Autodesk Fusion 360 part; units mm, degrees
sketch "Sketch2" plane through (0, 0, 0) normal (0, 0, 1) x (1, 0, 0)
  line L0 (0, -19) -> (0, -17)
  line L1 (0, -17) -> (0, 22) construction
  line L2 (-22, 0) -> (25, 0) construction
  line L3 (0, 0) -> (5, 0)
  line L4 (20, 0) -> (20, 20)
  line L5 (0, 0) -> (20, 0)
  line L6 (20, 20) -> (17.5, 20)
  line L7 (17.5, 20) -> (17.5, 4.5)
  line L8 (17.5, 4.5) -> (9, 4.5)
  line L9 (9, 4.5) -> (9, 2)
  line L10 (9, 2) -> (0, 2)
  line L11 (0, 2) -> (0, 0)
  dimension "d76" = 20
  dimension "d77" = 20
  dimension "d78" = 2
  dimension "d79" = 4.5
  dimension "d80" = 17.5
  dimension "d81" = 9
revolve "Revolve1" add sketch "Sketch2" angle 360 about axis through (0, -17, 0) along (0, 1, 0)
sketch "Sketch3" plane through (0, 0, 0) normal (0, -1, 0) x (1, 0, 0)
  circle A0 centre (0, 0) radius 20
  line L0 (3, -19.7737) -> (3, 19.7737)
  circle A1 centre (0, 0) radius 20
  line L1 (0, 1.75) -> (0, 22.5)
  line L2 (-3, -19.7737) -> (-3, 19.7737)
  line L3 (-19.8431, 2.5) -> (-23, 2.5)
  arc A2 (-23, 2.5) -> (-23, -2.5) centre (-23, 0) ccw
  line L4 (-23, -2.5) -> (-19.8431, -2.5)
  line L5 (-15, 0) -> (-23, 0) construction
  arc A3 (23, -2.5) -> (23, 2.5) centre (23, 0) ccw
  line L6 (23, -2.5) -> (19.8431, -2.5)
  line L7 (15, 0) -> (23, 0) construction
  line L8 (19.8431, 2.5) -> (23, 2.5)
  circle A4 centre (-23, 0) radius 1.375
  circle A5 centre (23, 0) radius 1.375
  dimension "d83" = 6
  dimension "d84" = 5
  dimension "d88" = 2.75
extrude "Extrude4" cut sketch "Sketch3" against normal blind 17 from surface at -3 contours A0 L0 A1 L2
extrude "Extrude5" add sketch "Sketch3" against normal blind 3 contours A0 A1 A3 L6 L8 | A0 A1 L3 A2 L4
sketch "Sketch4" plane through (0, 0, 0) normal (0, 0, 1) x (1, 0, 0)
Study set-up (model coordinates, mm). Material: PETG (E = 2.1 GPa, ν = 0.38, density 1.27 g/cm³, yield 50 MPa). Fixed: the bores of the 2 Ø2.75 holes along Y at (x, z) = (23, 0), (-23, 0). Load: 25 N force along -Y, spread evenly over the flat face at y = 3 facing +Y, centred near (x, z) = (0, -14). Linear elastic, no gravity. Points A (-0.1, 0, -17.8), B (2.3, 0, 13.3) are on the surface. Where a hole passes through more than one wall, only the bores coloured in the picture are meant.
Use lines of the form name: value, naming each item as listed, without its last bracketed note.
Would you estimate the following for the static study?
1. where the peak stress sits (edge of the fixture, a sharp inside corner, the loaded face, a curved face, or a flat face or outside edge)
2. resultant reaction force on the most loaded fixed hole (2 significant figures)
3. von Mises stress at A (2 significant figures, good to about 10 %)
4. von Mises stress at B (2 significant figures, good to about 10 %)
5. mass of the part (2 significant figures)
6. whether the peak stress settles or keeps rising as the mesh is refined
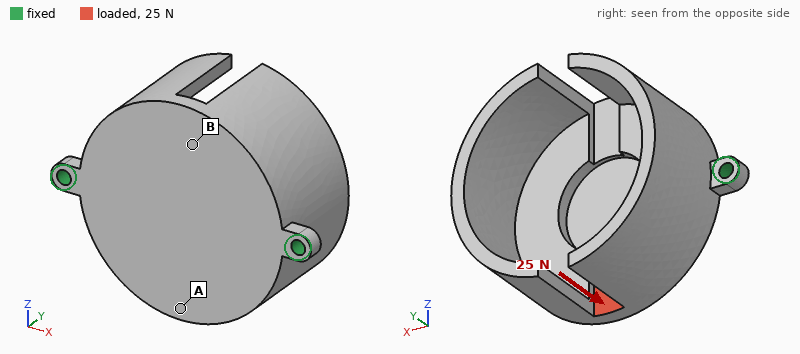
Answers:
where the peak stress sits: edge of the fixture
resultant reaction force on the most loaded fixed hole: 13 N
von Mises stress at A: 5.9 MPa
von Mises stress at B: 2.6 MPa
mass of the part: 11 g
whether the peak stress settles or keeps rising as the mesh is refined: keeps rising
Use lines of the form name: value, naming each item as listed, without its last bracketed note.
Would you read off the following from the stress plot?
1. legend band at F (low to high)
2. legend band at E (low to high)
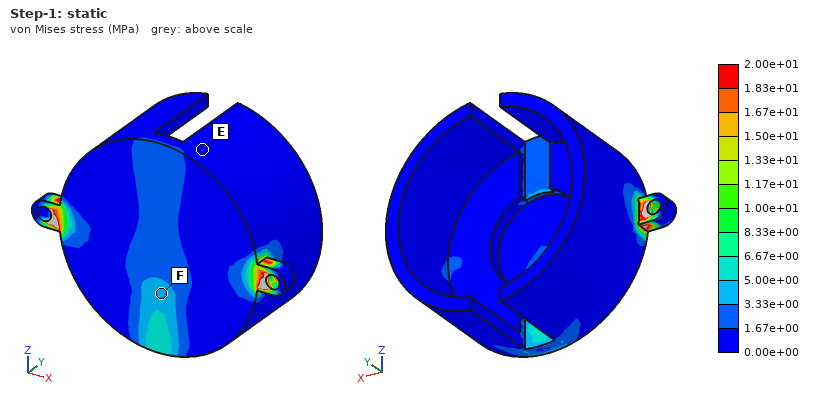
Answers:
legend band at F: 3.33e+00 to 5.00e+00 MPa
legend band at E: 0.00e+00 to 1.67e+00 MPa
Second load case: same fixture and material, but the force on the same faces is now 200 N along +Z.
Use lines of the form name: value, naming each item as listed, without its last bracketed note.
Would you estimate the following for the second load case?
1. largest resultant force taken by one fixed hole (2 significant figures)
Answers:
largest resultant force taken by one fixed hole: 100 N
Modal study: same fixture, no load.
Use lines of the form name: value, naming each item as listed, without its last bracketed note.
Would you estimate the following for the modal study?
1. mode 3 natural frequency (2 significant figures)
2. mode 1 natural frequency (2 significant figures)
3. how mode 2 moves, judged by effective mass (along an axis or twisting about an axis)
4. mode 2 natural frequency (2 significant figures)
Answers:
mode 3 natural frequency: 1400 Hz
mode 1 natural frequency: 430 Hz
how mode 2 moves, judged by effective mass: along Y
mode 2 natural frequency: 840 Hz
